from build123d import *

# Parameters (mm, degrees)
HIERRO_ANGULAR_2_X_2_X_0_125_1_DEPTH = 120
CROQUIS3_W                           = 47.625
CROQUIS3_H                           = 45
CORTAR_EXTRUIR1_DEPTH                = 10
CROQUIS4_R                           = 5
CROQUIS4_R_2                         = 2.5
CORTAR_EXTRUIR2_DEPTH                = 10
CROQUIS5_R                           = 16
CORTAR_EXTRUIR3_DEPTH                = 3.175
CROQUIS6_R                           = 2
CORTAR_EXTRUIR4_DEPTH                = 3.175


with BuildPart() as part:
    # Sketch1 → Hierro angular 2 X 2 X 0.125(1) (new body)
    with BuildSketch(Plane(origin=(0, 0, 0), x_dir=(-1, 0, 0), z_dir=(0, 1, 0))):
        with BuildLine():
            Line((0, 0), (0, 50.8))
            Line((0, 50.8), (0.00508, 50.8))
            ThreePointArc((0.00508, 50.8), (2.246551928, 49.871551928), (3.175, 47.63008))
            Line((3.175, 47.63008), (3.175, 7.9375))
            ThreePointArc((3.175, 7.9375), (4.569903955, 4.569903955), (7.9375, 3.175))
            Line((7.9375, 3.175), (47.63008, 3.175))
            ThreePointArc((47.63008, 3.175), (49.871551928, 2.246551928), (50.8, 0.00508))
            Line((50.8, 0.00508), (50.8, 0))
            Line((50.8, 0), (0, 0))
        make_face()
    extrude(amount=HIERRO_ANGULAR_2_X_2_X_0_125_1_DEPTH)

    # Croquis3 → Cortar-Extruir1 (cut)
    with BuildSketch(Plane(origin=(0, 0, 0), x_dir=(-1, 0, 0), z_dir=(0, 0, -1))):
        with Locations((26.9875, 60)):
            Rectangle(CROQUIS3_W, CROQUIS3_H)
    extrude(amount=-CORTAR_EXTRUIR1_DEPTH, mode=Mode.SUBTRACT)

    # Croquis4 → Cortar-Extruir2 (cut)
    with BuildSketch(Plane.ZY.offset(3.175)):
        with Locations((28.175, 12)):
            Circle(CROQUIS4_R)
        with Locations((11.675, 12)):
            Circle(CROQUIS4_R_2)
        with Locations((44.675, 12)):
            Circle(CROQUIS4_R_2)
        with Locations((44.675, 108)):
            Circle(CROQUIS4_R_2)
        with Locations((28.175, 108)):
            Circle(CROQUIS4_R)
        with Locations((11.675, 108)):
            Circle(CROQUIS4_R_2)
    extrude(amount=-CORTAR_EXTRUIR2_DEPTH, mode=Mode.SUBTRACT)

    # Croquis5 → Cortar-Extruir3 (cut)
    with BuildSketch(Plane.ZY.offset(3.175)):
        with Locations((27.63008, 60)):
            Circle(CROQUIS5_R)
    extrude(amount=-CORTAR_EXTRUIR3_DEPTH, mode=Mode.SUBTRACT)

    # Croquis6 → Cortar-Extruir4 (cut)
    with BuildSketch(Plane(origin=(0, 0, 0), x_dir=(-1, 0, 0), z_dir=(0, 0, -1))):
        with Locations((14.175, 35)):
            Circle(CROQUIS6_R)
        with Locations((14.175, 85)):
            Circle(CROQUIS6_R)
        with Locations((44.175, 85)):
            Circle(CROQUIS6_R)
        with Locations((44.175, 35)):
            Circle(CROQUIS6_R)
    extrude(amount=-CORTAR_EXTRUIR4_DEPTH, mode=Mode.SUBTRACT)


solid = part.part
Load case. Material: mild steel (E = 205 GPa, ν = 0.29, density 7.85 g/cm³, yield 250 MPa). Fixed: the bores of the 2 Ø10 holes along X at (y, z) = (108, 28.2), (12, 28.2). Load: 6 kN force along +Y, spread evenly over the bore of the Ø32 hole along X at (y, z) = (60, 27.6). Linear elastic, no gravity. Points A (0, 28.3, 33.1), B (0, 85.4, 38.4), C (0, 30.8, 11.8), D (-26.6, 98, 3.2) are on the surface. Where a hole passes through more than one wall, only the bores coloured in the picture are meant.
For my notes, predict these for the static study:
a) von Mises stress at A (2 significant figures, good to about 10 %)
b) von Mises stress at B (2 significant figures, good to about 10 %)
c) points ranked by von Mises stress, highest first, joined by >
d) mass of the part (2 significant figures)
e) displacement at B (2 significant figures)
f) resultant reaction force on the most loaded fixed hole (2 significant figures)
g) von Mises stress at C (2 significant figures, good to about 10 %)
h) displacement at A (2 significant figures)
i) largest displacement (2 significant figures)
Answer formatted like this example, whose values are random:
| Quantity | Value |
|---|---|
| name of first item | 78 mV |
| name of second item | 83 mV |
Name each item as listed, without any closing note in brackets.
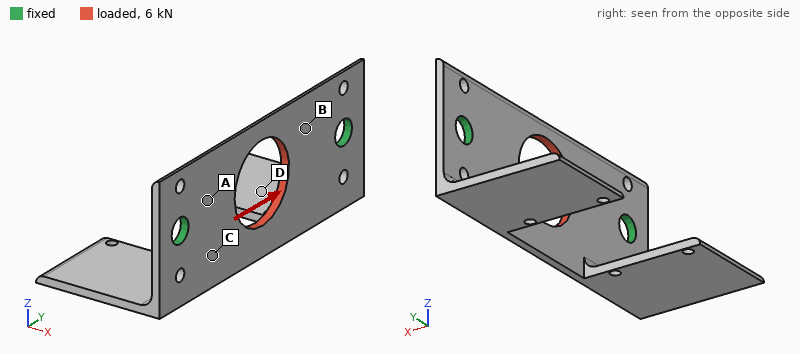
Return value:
| Quantity | Value |
|---|---|
| von Mises stress at A | 31 MPa |
| von Mises stress at B | 25 MPa |
| points ranked by von Mises stress, highest first, joined by > | A > B > C > D |
| mass of the part | 210 g |
| displacement at B | 3.4 µm |
| resultant reaction force on the most loaded fixed hole | 3.0 kN |
| von Mises stress at C | 18 MPa |
| displacement at A | 2.3 µm |
| largest displacement | 6.4 µm |
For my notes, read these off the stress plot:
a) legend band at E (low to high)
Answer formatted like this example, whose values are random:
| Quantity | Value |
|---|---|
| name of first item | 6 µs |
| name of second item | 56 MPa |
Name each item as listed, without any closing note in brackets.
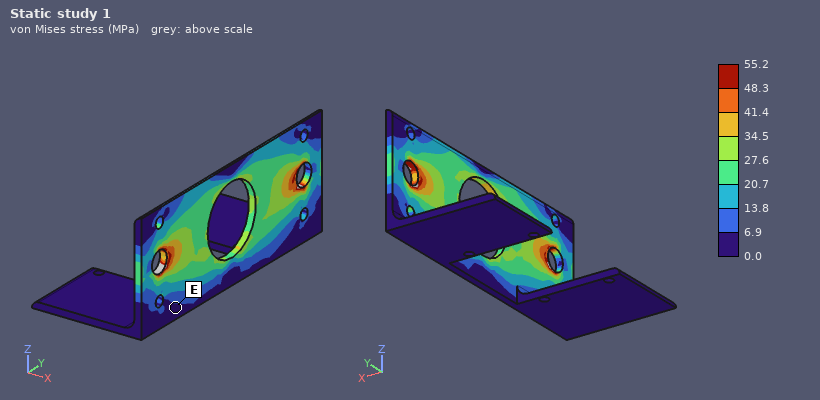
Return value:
| Quantity | Value |
|---|---|
| legend band at E | 0.0 to 6.9 MPa |
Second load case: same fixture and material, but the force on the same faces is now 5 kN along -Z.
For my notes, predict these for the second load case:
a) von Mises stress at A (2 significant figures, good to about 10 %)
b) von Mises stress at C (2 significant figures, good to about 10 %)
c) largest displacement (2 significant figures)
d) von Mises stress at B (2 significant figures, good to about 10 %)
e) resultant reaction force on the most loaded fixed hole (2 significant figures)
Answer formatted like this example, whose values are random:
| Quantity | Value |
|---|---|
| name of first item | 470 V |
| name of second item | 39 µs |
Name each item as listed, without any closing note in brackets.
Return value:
| Quantity | Value |
|---|---|
| von Mises stress at A | 38 MPa |
| von Mises stress at C | 33 MPa |
| largest displacement | 22 µm |
| von Mises stress at B | 33 MPa |
| resultant reaction force on the most loaded fixed hole | 2.5 kN |
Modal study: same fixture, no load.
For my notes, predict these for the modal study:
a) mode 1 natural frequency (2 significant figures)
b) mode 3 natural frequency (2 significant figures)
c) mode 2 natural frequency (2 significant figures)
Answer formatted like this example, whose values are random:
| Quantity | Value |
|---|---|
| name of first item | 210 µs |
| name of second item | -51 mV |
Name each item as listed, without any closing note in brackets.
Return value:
| Quantity | Value |
|---|---|
| mode 1 natural frequency | 660 Hz |
| mode 3 natural frequency | 1100 Hz |
| mode 2 natural frequency | 750 Hz |
